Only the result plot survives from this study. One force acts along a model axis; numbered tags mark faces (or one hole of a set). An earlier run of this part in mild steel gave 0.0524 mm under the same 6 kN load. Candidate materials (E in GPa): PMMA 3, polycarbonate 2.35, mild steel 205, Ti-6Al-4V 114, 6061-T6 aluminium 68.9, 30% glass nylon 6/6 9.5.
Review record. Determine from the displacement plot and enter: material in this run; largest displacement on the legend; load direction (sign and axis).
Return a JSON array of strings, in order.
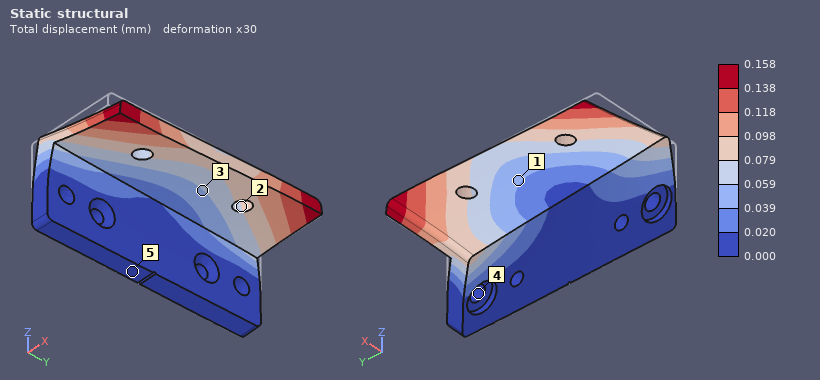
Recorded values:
["6061-T6 aluminium", "0.158 mm", "+Y"]
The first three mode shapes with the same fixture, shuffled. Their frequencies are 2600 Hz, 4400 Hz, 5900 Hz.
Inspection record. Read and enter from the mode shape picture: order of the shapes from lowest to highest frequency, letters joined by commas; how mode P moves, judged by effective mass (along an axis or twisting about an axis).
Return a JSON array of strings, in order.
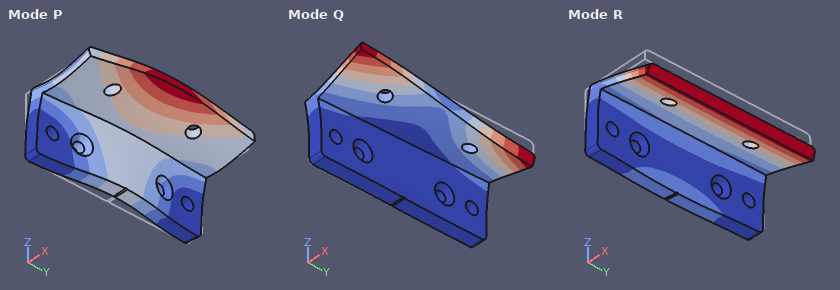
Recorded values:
["R, Q, P", "along X"]
